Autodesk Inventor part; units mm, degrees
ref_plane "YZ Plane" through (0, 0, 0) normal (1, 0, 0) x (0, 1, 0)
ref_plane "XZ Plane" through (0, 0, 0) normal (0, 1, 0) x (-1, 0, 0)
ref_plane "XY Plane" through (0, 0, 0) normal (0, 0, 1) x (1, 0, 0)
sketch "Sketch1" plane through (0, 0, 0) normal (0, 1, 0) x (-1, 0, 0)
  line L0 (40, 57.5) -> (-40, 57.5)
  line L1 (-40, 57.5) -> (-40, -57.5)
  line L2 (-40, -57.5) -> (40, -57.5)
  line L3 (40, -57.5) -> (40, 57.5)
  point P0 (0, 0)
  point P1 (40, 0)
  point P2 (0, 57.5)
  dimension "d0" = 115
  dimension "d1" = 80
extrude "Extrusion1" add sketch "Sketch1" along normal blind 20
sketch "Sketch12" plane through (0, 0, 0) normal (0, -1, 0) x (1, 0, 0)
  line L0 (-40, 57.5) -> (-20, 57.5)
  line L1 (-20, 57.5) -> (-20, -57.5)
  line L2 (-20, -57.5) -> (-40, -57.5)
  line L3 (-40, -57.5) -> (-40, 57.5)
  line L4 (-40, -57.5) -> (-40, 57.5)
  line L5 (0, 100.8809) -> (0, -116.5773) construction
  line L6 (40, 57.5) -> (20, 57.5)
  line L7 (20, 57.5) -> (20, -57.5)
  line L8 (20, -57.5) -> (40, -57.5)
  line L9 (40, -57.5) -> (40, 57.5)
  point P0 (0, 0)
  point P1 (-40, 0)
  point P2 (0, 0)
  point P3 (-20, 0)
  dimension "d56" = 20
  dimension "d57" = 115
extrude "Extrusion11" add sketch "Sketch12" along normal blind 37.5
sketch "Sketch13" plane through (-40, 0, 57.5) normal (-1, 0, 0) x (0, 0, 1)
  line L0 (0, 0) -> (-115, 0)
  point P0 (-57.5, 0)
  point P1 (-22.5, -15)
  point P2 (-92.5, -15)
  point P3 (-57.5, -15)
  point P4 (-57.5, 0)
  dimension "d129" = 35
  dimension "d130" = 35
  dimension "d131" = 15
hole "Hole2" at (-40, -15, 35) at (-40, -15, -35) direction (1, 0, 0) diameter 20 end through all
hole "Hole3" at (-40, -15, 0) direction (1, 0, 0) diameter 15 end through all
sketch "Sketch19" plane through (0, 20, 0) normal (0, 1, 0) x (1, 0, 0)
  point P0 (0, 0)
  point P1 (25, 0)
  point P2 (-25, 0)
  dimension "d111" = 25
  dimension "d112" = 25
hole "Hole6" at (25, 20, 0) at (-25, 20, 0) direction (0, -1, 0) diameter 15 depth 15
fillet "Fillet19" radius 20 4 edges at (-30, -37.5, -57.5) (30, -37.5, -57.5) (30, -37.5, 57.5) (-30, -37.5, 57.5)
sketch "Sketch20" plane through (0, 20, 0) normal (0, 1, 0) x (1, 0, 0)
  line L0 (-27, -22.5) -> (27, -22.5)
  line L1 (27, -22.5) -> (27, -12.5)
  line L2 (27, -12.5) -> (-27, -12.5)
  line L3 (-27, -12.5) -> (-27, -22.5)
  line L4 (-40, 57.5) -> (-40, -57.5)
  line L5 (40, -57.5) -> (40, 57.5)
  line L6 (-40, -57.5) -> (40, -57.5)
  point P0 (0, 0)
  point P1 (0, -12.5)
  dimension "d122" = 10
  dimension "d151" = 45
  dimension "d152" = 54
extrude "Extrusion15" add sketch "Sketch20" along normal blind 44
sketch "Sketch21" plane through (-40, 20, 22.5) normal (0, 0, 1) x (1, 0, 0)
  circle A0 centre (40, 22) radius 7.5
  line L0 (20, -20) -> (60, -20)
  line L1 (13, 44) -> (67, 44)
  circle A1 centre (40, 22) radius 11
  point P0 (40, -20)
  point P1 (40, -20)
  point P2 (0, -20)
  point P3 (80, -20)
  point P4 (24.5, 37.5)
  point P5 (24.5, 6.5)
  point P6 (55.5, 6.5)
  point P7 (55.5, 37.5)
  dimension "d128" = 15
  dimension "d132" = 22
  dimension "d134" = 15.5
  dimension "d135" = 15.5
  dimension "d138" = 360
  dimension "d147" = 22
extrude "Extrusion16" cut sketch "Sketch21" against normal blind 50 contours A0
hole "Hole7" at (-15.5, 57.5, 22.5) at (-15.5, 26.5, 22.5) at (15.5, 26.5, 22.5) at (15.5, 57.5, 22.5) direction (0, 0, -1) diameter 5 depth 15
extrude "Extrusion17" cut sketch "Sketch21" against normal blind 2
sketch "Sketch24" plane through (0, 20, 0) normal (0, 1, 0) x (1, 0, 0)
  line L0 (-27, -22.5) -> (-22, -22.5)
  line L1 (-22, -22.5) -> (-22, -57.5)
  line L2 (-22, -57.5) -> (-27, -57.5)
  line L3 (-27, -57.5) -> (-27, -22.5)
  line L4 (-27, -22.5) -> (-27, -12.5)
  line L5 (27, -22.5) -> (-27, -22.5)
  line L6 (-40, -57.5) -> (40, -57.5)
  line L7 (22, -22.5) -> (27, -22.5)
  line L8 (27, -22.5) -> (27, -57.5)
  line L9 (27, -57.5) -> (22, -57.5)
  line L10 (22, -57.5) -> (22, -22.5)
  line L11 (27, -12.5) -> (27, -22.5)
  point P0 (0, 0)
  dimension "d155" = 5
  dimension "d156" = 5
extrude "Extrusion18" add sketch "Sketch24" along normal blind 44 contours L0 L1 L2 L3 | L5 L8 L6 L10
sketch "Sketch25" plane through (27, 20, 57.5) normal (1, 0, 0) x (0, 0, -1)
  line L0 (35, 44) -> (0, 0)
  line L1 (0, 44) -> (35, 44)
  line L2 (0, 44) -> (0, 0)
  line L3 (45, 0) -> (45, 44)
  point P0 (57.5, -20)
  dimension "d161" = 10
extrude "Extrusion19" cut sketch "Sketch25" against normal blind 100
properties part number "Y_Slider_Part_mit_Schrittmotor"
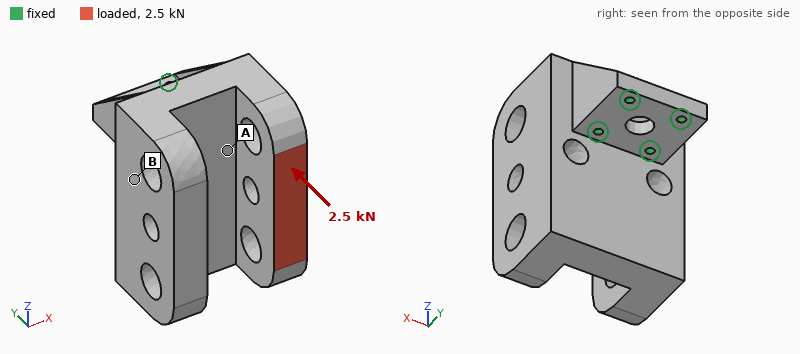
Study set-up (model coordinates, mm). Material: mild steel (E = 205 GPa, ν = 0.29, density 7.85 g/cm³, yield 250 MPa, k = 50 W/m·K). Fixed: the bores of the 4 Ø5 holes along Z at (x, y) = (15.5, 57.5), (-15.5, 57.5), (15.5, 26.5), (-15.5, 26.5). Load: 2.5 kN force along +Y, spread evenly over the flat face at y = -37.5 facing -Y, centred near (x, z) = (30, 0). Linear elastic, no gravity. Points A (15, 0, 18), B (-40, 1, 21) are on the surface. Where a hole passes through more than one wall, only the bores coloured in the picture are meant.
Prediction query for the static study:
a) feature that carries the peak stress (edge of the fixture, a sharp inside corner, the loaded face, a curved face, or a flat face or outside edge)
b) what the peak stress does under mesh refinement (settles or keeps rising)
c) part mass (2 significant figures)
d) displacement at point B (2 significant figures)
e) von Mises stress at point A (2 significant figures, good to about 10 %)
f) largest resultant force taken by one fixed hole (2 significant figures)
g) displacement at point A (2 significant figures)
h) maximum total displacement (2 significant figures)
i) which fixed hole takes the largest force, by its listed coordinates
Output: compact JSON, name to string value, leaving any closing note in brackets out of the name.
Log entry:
{"feature that carries the peak stress": "edge of the fixture", "what the peak stress does under mesh refinement": "keeps rising", "part mass": "2.7 kg", "displacement at point B": "3.8 µm", "von Mises stress at point A": "6.4 MPa", "largest resultant force taken by one fixed hole": "3.0 kN", "displacement at point A": "4.3 µm", "maximum total displacement": "21 µm", "which fixed hole takes the largest force, by its listed coordinates": "(15.5, 26.5)"}
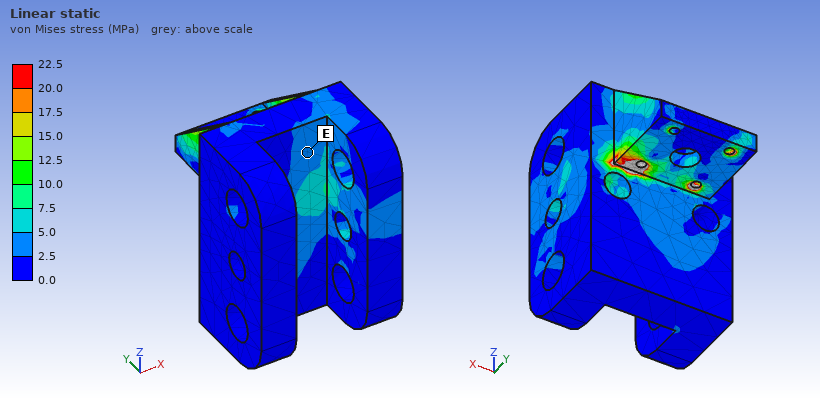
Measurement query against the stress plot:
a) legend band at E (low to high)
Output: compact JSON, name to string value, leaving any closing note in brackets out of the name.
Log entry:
{"legend band at E": "2.5 to 5.0 MPa"}
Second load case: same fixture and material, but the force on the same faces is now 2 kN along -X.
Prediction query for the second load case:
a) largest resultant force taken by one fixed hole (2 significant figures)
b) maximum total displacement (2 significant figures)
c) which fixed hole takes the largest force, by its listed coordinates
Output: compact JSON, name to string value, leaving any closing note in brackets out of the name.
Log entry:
{"largest resultant force taken by one fixed hole": "3.5 kN", "maximum total displacement": "22 µm", "which fixed hole takes the largest force, by its listed coordinates": "(-15.5, 26.5)"}
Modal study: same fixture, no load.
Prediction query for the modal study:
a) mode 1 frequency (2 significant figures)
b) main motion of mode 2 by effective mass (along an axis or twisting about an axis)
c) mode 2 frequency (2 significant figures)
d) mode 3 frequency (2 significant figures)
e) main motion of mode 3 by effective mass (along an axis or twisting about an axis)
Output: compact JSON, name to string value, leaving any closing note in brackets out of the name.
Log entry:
{"mode 1 frequency": "1100 Hz", "main motion of mode 2 by effective mass": "along X", "mode 2 frequency": "1800 Hz", "mode 3 frequency": "2500 Hz", "main motion of mode 3 by effective mass": "along X"}
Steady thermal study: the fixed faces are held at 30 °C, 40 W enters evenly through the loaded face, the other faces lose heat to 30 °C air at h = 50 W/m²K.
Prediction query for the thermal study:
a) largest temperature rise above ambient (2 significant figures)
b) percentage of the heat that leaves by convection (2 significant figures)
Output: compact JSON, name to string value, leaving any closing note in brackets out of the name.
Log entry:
{"largest temperature rise above ambient": "34 K", "percentage of the heat that leaves by convection": "63 %"}
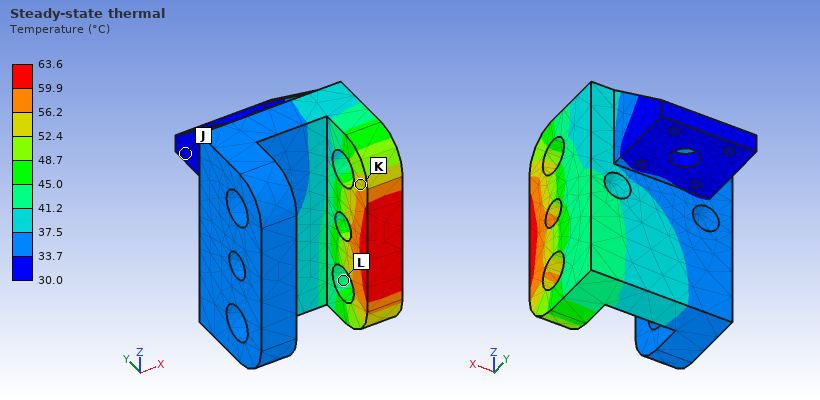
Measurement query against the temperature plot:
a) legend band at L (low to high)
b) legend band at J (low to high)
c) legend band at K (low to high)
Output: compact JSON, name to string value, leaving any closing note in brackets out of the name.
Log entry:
{"legend band at L": "41.2 to 45.0 °C", "legend band at J": "30.0 to 33.7 °C", "legend band at K": "52.4 to 56.2 °C"}
